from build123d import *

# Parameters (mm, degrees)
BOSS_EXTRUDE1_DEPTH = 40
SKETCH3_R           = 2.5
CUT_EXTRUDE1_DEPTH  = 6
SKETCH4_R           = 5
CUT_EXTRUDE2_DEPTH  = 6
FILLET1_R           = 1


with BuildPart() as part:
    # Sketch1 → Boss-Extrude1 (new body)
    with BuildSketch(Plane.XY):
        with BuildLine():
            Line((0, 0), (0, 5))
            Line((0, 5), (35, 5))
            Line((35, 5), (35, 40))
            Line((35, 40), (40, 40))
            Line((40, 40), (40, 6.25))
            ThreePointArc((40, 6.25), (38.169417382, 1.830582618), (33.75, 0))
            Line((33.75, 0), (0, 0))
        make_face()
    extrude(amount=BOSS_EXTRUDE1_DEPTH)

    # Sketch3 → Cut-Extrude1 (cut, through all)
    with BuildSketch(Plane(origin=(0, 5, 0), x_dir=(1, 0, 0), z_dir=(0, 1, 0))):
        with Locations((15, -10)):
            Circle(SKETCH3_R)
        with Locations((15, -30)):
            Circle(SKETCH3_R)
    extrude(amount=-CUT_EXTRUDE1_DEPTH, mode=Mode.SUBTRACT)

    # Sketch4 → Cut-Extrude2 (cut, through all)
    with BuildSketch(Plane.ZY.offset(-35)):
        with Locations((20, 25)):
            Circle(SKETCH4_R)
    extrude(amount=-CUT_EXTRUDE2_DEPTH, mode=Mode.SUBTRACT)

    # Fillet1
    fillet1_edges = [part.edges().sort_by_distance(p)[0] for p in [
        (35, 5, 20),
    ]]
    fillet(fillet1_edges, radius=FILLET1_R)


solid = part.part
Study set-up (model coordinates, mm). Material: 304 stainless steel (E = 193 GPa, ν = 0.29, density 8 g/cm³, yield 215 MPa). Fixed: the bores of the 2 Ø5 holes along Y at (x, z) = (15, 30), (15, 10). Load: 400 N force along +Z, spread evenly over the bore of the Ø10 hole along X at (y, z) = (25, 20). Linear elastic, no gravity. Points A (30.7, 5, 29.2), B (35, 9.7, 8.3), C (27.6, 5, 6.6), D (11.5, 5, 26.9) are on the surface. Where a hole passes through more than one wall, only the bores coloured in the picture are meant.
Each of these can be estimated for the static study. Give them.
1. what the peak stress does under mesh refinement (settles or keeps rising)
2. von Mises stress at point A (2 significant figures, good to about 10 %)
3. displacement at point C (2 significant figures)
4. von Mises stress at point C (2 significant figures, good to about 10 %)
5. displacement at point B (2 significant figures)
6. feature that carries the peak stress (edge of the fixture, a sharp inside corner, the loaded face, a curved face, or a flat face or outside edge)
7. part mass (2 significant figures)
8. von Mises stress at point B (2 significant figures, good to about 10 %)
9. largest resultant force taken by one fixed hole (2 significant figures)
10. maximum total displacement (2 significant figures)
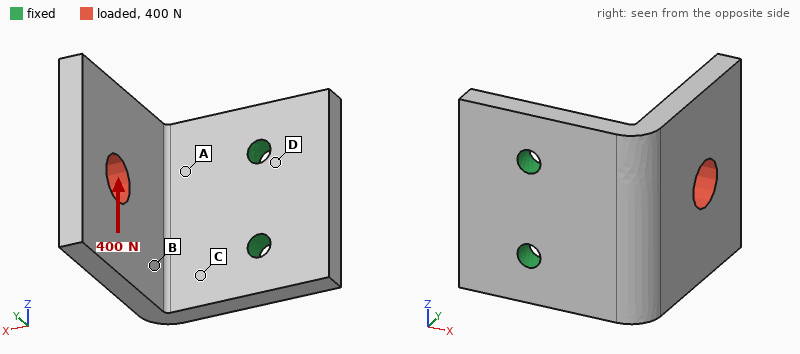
keeps rising
32 MPa
5.9 µm
28 MPa
12 µm
edge of the fixture
110 g
19 MPa
540 N
38 µm
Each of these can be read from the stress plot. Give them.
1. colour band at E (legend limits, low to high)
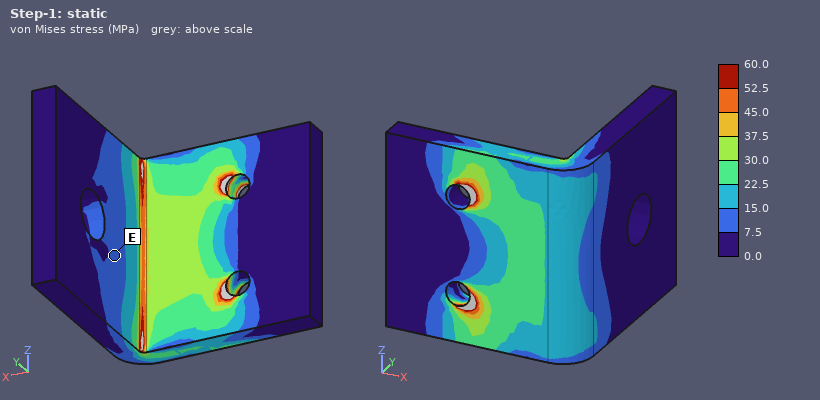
7.5 to 15.0 MPa
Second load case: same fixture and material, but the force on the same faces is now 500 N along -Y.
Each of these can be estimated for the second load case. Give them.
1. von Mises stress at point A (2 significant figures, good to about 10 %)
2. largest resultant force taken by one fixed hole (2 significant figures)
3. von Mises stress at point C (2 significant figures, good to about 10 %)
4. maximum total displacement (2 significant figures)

18 MPa
250 N
27 MPa
61 µm
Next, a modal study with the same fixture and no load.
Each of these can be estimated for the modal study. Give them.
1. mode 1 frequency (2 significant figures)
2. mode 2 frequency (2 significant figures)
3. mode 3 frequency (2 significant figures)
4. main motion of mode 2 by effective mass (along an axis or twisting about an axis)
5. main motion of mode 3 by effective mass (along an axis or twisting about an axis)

1500 Hz
2700 Hz
4600 Hz
along Z
along Y
